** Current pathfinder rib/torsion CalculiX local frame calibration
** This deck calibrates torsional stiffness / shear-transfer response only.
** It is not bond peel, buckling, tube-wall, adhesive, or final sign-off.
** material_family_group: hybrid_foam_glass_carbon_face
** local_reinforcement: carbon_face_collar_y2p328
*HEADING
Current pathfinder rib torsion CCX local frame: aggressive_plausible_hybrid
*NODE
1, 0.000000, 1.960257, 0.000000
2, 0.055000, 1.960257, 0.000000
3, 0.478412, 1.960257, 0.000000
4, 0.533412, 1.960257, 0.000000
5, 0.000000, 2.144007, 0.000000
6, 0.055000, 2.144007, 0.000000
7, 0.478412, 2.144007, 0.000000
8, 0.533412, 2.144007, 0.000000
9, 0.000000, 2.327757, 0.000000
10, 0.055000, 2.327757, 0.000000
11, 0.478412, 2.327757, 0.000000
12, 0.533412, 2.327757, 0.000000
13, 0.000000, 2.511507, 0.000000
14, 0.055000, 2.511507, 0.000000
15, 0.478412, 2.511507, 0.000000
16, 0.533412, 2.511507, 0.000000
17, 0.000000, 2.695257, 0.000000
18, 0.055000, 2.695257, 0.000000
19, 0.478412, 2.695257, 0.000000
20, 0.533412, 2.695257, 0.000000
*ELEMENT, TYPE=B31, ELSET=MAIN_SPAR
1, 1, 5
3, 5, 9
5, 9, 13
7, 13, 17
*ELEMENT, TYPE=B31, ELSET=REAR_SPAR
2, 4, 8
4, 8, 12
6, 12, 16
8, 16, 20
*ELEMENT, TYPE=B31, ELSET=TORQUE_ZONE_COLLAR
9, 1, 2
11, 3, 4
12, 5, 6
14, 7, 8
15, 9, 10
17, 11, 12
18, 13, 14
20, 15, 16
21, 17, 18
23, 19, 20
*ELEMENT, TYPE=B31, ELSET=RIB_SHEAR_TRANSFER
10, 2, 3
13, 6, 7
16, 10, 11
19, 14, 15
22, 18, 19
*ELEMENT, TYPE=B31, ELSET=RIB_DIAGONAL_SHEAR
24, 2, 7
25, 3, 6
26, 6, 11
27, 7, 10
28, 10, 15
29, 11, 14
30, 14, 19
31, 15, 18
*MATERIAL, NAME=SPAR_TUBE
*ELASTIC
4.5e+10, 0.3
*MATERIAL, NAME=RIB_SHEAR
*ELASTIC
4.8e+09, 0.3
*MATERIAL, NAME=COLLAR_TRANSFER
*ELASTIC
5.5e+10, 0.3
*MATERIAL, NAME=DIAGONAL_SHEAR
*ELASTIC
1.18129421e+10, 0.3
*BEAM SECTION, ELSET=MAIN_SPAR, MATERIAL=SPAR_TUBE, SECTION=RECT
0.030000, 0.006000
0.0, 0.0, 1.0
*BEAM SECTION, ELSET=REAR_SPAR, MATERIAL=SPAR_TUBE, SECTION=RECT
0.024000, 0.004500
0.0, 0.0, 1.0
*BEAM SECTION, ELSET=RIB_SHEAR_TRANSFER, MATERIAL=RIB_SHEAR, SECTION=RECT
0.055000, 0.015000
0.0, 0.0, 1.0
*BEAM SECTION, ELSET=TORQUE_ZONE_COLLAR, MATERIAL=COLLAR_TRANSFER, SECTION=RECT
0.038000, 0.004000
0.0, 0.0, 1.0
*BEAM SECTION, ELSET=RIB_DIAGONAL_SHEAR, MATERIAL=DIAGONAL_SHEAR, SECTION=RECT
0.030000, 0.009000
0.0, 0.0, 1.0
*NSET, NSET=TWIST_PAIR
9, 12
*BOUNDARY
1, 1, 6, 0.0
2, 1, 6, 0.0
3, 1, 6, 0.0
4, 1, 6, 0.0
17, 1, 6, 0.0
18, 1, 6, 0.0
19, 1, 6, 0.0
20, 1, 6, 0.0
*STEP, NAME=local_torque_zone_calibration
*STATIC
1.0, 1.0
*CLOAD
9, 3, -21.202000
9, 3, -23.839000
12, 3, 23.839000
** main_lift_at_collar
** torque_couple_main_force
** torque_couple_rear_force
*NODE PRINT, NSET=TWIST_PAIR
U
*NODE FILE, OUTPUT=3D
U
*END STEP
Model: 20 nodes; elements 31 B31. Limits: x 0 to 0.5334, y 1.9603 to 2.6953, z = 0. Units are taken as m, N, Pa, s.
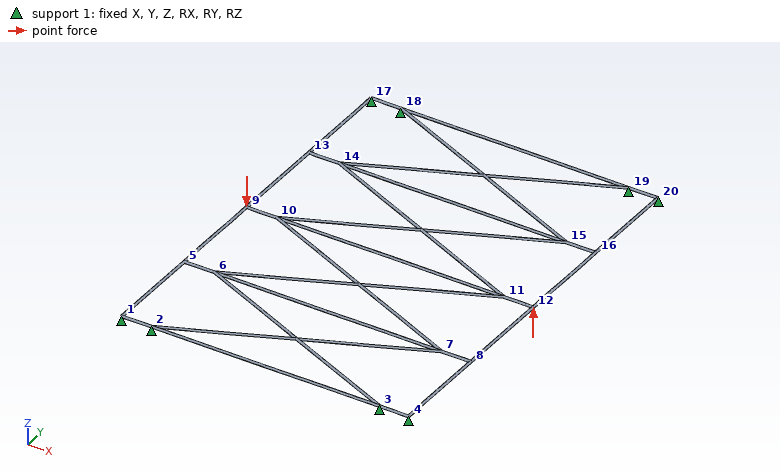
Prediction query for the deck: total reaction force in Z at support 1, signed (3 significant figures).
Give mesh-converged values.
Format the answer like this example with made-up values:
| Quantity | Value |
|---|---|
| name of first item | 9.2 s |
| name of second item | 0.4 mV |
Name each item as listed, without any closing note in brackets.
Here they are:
| Quantity | Value |
|---|---|
| total reaction force in Z at support 1, signed | 21.2 N |
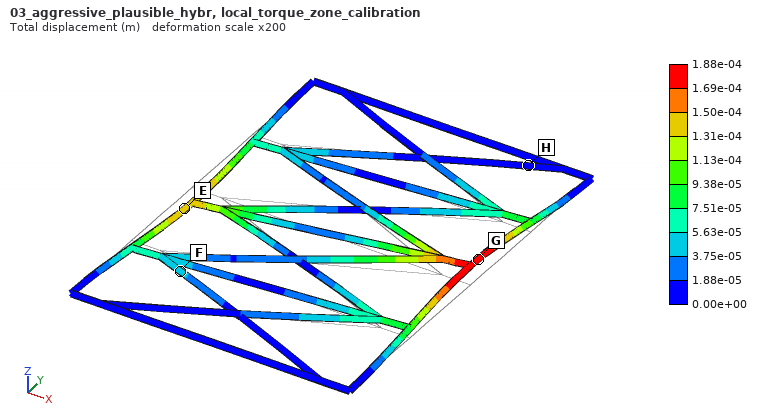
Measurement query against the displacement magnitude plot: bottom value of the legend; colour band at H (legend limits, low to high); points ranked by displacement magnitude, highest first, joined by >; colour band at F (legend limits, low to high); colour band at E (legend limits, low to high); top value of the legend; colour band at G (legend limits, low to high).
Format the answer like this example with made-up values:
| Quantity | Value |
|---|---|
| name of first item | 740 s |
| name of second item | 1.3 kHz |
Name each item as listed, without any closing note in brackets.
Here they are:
| Quantity | Value |
|---|---|
| bottom value of the legend | 0.00e+00 m |
| colour band at H | 0.00e+00 to 1.88e-05 m |
| points ranked by displacement magnitude, highest first, joined by > | G > E > F > H |
| colour band at F | 3.75e-05 to 5.63e-05 m |
| colour band at E | 1.31e-04 to 1.50e-04 m |
| top value of the legend | 1.88e-04 m |
| colour band at G | 1.69e-04 to 1.88e-04 m |
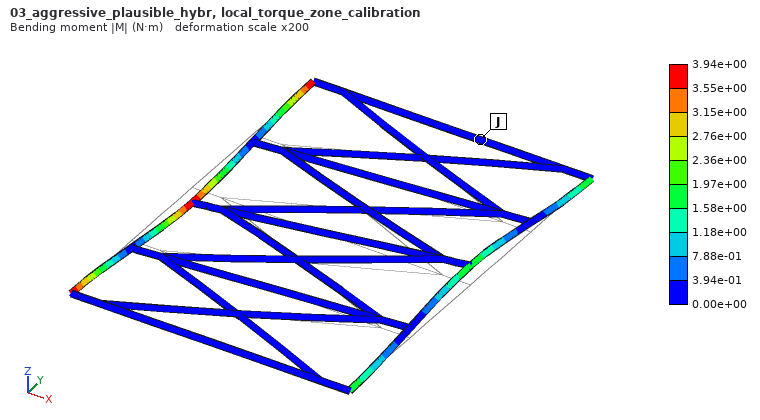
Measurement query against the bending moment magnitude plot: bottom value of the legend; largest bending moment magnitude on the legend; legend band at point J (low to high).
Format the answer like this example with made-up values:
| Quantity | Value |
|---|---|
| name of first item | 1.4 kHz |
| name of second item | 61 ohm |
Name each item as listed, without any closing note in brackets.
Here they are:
| Quantity | Value |
|---|---|
| bottom value of the legend | 0.00e+00 N·m |
| largest bending moment magnitude on the legend | 3.94e+00 N·m |
| legend band at point J | 0.00e+00 to 3.94e-01 N·m |
